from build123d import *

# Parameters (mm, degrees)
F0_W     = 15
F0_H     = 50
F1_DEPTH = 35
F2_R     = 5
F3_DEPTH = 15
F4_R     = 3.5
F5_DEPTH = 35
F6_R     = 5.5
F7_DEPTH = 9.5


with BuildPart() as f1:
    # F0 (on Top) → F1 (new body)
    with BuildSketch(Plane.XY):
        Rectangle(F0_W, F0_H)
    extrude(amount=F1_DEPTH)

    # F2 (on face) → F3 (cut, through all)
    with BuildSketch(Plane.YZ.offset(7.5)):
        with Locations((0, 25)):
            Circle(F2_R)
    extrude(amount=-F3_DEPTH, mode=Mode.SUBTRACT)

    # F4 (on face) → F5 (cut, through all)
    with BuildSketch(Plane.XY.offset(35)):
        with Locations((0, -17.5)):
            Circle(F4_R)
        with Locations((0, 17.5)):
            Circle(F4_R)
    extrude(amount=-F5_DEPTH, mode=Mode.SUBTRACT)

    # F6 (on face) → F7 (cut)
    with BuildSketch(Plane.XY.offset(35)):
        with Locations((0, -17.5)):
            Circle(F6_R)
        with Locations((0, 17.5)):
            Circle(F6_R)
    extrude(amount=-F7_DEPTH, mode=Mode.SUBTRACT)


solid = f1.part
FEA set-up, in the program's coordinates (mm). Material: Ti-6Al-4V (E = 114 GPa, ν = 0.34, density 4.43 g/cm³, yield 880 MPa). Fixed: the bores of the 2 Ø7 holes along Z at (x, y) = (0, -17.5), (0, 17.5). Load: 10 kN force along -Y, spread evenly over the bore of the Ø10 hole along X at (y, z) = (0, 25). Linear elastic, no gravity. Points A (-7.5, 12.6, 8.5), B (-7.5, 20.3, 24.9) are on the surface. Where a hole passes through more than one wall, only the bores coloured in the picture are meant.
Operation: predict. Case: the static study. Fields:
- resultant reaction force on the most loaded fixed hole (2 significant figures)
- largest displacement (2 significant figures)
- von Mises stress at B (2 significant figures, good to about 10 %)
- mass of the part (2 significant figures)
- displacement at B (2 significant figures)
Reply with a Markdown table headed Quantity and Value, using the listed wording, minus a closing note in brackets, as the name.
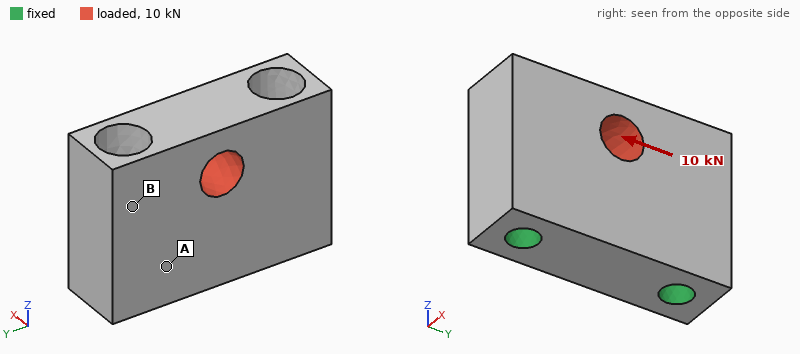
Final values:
| Quantity | Value |
|---|---|
| resultant reaction force on the most loaded fixed hole | 5.2 kN |
| largest displacement | 5.9 µm |
| von Mises stress at B | 18 MPa |
| mass of the part | 94 g |
| displacement at B | 1.3 µm |
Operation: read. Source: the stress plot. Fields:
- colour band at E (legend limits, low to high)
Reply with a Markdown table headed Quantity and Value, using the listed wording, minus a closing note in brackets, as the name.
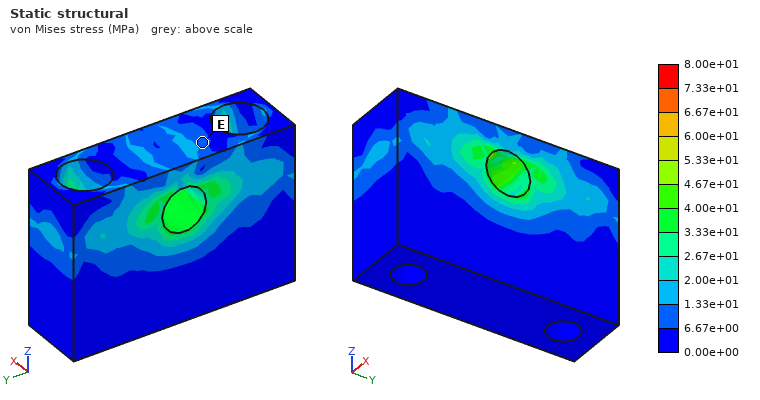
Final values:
| Quantity | Value |
|---|---|
| colour band at E | 6.67e+00 to 1.33e+01 MPa |
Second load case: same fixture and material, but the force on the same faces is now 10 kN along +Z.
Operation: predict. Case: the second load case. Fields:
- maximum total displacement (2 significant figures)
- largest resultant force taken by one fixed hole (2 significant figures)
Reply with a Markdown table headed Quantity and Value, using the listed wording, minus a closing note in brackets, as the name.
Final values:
| Quantity | Value |
|---|---|
| maximum total displacement | 7.6 µm |
| largest resultant force taken by one fixed hole | 5.3 kN |
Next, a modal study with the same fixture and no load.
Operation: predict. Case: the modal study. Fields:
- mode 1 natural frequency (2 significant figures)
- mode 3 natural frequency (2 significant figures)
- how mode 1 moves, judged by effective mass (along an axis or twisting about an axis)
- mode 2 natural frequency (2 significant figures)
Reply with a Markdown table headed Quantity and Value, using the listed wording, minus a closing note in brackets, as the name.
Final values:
| Quantity | Value |
|---|---|
| mode 1 natural frequency | 25 kHz |
| mode 3 natural frequency | 38 kHz |
| how mode 1 moves, judged by effective mass | along X |
| mode 2 natural frequency | 38 kHz |
